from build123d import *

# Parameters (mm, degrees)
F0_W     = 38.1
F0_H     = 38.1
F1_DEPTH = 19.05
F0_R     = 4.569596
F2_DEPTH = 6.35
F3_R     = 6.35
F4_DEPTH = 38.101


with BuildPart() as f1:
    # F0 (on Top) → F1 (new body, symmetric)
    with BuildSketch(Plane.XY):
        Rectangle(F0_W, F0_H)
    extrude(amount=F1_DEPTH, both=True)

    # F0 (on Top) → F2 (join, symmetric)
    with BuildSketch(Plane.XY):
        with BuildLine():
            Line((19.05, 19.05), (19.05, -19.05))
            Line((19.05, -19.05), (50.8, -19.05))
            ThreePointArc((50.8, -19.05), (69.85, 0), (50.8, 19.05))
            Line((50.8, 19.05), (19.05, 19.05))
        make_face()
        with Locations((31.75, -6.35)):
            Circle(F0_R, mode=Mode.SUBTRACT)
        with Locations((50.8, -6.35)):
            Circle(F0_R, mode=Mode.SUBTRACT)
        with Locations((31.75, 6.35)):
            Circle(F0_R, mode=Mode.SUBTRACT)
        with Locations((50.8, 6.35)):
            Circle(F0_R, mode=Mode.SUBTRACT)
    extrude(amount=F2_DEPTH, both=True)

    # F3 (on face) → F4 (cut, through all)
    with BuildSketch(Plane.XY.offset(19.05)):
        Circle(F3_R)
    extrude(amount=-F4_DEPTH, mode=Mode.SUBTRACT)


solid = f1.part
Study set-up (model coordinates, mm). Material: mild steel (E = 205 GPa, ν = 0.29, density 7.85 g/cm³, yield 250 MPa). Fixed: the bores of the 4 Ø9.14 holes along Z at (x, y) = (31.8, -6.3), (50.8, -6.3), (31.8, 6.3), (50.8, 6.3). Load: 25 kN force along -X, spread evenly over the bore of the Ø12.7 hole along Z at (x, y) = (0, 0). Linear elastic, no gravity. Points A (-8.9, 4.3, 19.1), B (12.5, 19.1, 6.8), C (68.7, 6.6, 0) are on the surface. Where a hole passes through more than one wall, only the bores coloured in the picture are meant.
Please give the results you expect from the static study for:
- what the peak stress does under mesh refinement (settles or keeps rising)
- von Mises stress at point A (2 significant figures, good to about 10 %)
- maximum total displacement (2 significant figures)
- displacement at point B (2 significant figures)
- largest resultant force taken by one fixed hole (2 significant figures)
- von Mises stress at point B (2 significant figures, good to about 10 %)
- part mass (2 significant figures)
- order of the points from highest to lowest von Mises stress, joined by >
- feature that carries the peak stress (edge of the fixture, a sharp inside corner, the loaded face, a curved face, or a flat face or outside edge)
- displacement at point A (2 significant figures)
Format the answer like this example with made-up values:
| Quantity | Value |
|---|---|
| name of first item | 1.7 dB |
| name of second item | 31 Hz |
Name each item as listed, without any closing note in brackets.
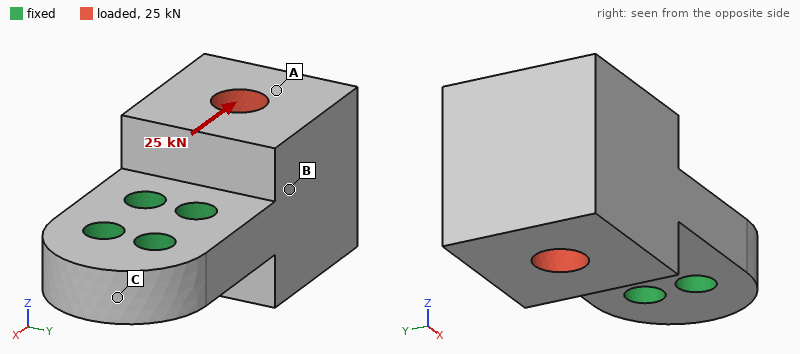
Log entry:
| Quantity | Value |
|---|---|
| what the peak stress does under mesh refinement | keeps rising |
| von Mises stress at point A | 18 MPa |
| maximum total displacement | 7.9 µm |
| displacement at point B | 4.5 µm |
| largest resultant force taken by one fixed hole | 12 kN |
| von Mises stress at point B | 28 MPa |
| part mass | 550 g |
| order of the points from highest to lowest von Mises stress, joined by > | B > A > C |
| feature that carries the peak stress | edge of the fixture |
| displacement at point A | 7.3 µm |
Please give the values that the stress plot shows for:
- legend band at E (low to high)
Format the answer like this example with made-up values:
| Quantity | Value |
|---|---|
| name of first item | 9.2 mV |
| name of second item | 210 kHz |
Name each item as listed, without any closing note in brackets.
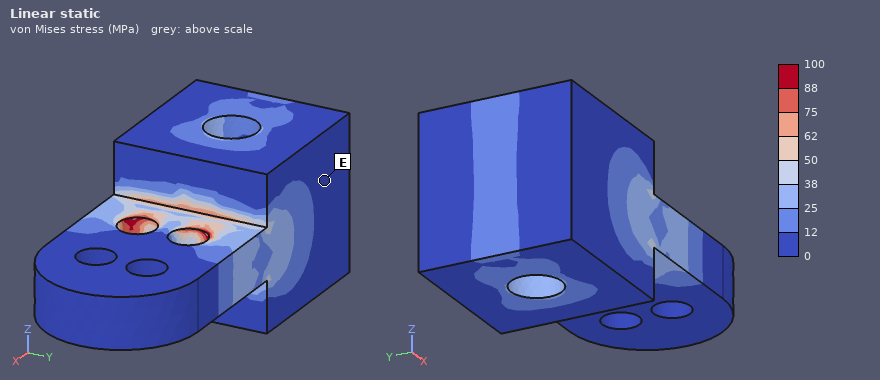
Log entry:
| Quantity | Value |
|---|---|
| legend band at E | 0 to 12 MPa |
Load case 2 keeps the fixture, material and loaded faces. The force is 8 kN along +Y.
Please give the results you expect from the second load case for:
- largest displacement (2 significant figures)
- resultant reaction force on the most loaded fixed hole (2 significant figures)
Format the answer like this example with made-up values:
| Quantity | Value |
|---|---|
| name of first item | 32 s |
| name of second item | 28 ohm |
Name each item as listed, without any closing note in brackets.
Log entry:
| Quantity | Value |
|---|---|
| largest displacement | 22 µm |
| resultant reaction force on the most loaded fixed hole | 9.9 kN |
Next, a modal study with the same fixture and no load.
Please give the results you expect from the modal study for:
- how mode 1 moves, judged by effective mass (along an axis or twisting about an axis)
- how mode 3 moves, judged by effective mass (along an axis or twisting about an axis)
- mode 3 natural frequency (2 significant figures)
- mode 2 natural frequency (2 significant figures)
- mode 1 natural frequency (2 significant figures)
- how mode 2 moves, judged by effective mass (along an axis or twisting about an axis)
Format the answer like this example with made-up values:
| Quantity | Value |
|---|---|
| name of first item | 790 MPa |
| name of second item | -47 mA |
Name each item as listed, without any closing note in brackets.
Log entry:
| Quantity | Value |
|---|---|
| how mode 1 moves, judged by effective mass | along Z |
| how mode 3 moves, judged by effective mass | twisting about X |
| mode 3 natural frequency | 7200 Hz |
| mode 2 natural frequency | 5500 Hz |
| mode 1 natural frequency | 2700 Hz |
| how mode 2 moves, judged by effective mass | along Y |
